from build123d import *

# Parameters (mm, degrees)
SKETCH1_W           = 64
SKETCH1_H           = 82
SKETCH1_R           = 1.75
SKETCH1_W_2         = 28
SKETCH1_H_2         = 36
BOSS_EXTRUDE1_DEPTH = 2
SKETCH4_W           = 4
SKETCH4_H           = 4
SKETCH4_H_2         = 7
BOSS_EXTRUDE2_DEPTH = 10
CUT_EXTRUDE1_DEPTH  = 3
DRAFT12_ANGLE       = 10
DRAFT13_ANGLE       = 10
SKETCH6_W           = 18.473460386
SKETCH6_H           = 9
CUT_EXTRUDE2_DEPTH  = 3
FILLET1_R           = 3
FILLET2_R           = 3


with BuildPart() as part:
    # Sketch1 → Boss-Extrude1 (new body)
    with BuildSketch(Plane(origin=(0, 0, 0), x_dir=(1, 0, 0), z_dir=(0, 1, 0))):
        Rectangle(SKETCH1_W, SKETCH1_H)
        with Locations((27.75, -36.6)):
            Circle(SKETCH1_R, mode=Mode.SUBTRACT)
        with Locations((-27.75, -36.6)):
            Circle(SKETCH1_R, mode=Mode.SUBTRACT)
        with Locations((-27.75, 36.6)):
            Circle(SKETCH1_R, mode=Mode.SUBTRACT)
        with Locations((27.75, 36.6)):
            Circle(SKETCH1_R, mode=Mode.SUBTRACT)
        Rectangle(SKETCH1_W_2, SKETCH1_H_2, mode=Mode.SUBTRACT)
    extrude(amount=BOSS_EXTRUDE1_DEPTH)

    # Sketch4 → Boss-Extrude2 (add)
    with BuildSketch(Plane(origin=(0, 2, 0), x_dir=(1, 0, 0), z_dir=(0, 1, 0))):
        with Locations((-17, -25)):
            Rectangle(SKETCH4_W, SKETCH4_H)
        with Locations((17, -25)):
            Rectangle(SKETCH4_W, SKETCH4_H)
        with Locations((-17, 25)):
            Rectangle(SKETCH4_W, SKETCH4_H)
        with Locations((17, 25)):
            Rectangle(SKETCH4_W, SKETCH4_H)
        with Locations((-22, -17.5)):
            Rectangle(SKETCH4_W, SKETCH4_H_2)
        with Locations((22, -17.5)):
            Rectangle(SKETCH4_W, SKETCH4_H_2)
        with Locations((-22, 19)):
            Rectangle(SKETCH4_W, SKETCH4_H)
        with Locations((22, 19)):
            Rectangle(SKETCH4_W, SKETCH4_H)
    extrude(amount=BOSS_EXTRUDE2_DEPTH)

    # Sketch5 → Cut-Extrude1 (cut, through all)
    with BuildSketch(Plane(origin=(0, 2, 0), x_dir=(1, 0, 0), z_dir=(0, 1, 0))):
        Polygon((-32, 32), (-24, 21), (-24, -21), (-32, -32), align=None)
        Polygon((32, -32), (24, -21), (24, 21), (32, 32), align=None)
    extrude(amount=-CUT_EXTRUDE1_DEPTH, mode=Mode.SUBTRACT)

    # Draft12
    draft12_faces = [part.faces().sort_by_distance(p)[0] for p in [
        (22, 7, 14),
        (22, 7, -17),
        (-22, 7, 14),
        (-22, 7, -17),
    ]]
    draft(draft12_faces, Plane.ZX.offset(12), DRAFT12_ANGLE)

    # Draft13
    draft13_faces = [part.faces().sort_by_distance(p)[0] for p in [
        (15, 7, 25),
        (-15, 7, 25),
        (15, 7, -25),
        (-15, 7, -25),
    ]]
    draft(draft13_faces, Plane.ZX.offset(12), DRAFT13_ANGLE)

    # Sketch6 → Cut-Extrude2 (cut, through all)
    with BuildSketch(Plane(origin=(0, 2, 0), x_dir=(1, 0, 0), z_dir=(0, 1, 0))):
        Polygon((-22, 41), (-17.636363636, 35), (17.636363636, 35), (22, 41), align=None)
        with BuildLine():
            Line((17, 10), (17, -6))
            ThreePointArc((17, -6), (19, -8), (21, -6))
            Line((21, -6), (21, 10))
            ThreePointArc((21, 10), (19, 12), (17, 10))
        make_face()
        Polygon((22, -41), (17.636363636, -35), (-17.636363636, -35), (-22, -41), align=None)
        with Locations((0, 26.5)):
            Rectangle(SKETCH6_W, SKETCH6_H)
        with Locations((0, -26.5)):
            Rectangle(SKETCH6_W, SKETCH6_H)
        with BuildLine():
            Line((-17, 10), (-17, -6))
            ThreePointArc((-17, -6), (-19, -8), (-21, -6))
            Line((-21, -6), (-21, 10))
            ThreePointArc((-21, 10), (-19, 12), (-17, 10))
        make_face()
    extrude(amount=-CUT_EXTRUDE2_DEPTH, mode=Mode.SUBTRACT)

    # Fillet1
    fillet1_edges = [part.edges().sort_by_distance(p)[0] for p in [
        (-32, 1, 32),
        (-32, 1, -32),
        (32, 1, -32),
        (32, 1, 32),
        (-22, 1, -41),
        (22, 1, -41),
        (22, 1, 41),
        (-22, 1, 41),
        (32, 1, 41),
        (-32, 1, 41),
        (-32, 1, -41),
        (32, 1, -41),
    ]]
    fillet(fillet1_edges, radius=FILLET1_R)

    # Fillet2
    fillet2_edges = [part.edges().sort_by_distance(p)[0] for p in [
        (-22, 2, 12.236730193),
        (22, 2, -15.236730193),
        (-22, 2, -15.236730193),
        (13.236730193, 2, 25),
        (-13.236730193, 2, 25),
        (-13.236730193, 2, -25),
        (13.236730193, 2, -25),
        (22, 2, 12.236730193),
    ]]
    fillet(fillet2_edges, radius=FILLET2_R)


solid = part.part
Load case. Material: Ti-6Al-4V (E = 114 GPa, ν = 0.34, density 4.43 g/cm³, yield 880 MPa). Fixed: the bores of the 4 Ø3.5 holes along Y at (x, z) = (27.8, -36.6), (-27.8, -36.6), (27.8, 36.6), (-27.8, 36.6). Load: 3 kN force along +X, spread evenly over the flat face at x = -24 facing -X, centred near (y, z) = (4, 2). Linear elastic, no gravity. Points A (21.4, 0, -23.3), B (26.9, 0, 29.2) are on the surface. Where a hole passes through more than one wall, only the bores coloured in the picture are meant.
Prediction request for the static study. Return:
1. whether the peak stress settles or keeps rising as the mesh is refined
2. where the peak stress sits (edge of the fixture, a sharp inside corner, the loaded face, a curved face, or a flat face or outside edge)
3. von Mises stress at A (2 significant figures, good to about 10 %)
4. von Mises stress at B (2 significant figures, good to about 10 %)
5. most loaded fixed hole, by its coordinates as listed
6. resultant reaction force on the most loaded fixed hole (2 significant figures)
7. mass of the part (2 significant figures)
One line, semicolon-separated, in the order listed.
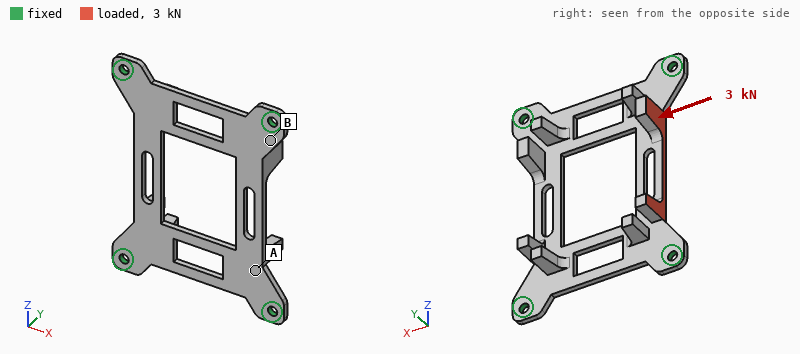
keeps rising; a sharp inside corner; 77 MPa; 170 MPa; (-27.8, 36.6); 1.3 kN; 29 g
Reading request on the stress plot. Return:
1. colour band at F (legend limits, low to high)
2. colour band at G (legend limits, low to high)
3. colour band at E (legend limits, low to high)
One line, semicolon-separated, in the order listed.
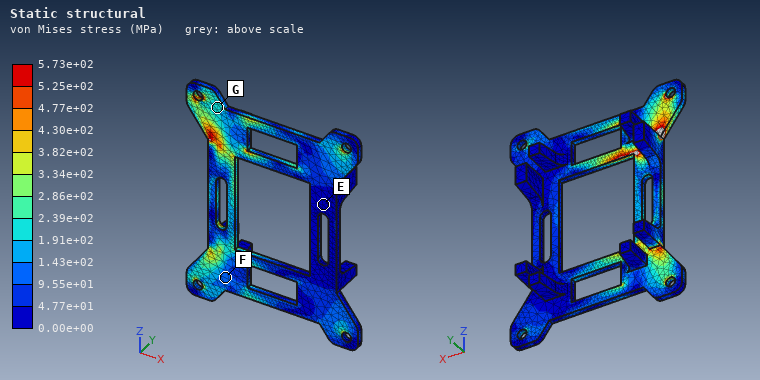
9.55e+01 to 1.43e+02 MPa; 1.91e+02 to 2.39e+02 MPa; 0.00e+00 to 4.77e+01 MPa
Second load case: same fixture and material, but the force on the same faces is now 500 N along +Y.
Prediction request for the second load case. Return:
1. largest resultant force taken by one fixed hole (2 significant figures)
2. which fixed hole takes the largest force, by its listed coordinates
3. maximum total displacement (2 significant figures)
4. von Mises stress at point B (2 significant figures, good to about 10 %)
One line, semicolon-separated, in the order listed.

260 N; (-27.8, 36.6); 0.74 mm; 50 MPa
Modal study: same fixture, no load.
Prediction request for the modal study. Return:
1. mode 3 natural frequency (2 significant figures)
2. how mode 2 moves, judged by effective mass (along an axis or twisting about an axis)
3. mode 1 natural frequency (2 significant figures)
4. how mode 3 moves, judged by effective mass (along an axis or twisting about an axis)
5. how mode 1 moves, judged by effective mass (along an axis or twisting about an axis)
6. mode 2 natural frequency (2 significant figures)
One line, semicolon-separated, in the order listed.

2900 Hz; twisting about Z; 1600 Hz; twisting about X; along Y; 2200 Hz
